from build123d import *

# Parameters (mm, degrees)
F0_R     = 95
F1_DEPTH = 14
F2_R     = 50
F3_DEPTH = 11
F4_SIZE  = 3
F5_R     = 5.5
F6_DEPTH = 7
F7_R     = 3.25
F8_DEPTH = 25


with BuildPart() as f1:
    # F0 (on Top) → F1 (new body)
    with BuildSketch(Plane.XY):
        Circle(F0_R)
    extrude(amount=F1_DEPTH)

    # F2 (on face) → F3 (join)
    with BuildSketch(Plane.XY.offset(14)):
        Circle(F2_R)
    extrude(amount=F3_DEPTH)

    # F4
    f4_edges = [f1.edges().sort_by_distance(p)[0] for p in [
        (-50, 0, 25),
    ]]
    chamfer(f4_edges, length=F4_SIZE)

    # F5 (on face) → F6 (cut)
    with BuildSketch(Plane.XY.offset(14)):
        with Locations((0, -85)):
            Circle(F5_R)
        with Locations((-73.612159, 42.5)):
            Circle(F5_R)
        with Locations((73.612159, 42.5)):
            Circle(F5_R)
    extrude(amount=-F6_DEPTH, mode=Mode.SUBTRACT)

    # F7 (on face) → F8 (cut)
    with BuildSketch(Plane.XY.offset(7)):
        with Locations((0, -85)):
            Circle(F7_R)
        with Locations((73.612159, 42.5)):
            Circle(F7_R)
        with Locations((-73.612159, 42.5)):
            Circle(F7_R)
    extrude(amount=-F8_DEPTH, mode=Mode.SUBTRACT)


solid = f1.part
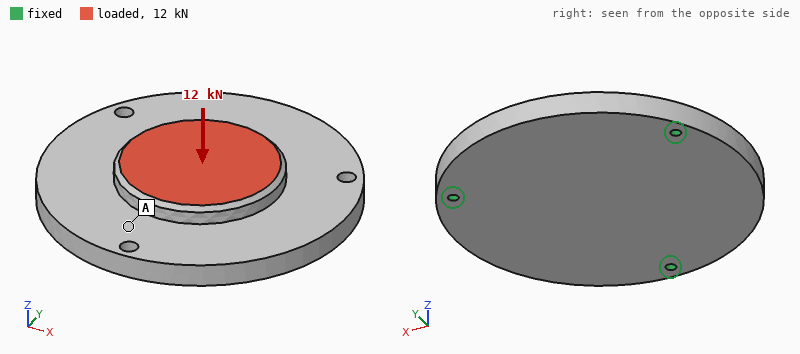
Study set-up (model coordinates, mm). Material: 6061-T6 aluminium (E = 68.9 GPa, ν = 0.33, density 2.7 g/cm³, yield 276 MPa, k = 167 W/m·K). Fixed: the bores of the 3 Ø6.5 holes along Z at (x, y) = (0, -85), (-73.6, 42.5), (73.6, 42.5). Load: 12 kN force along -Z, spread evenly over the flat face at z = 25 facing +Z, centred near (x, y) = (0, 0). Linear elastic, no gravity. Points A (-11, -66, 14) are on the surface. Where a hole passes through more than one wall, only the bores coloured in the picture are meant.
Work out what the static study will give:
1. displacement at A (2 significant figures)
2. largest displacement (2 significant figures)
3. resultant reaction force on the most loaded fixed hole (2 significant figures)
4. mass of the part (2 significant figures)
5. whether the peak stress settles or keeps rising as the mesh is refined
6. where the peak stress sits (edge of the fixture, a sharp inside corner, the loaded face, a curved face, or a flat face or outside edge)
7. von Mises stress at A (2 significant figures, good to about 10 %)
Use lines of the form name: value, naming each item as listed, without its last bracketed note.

displacement at A: 39 µm
largest displacement: 78 µm
resultant reaction force on the most loaded fixed hole: 5.9 kN
mass of the part: 1.3 kg
whether the peak stress settles or keeps rising as the mesh is refined: keeps rising
where the peak stress sits: edge of the fixture
von Mises stress at A: 20 MPa
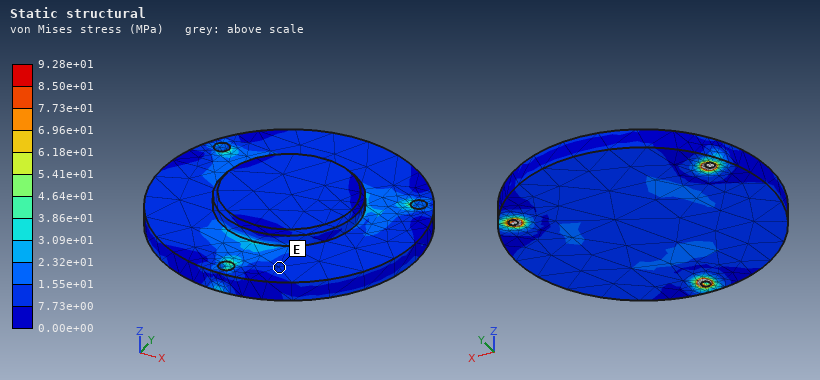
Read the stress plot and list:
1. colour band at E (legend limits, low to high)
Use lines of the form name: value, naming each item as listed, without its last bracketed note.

colour band at E: 7.73e+00 to 1.55e+01 MPa
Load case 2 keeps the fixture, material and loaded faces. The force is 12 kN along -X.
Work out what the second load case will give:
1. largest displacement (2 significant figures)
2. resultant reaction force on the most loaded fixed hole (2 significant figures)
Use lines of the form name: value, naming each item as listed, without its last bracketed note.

largest displacement: 44 µm
resultant reaction force on the most loaded fixed hole: 5.2 kN
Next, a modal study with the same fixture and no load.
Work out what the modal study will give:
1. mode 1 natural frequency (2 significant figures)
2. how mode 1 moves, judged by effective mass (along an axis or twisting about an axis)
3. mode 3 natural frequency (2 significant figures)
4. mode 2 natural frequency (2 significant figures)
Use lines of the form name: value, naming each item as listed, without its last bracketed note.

mode 1 natural frequency: 2100 Hz
how mode 1 moves, judged by effective mass: along Z
mode 3 natural frequency: 2200 Hz
mode 2 natural frequency: 2200 Hz
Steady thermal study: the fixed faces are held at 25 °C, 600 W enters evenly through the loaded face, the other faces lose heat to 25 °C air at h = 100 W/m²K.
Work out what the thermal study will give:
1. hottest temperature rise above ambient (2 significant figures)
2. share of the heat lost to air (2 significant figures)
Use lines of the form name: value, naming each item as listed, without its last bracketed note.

hottest temperature rise above ambient: 68 K
share of the heat lost to air: 40 %
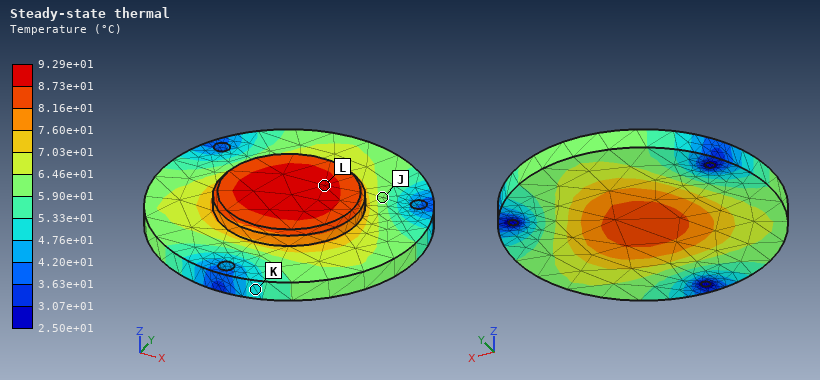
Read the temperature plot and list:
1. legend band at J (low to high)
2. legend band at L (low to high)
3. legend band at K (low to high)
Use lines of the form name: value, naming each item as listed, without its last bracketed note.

legend band at J: 5.90e+01 to 6.46e+01 °C
legend band at L: 8.73e+01 to 9.29e+01 °C
legend band at K: 4.76e+01 to 5.33e+01 °C
